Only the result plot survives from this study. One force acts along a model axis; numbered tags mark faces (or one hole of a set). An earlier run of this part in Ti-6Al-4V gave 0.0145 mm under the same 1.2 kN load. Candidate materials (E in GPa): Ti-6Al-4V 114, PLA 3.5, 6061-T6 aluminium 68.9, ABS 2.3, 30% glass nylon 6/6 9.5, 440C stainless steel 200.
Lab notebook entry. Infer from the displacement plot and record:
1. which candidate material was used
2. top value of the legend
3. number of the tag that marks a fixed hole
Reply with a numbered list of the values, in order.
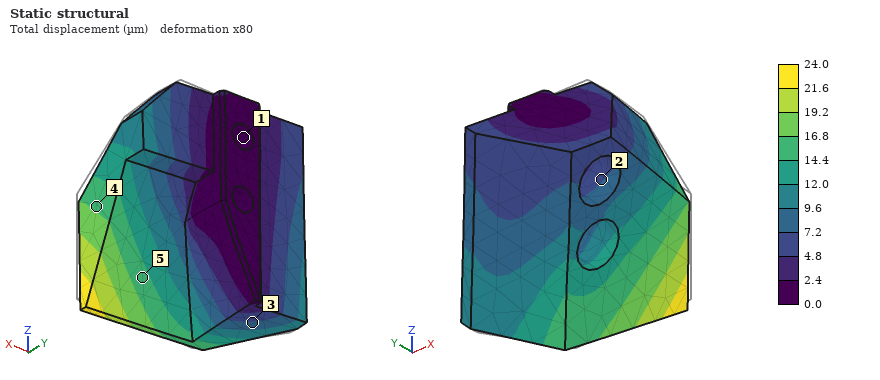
1. 6061-T6 aluminium
2. 24.0 µm
3. 1
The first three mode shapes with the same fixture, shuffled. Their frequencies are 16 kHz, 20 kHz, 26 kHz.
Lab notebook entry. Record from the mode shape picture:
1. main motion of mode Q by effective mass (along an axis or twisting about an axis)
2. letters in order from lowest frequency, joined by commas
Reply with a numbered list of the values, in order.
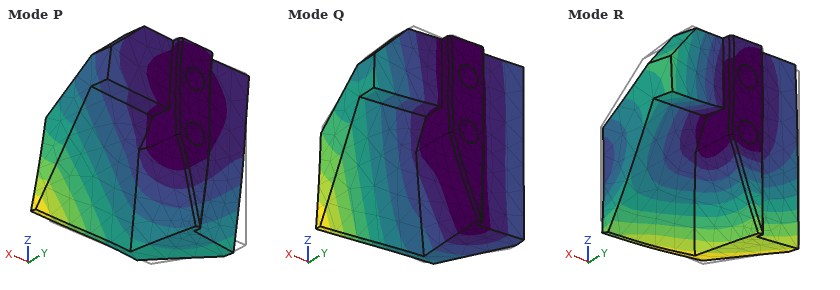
1. along X
2. Q, P, R
